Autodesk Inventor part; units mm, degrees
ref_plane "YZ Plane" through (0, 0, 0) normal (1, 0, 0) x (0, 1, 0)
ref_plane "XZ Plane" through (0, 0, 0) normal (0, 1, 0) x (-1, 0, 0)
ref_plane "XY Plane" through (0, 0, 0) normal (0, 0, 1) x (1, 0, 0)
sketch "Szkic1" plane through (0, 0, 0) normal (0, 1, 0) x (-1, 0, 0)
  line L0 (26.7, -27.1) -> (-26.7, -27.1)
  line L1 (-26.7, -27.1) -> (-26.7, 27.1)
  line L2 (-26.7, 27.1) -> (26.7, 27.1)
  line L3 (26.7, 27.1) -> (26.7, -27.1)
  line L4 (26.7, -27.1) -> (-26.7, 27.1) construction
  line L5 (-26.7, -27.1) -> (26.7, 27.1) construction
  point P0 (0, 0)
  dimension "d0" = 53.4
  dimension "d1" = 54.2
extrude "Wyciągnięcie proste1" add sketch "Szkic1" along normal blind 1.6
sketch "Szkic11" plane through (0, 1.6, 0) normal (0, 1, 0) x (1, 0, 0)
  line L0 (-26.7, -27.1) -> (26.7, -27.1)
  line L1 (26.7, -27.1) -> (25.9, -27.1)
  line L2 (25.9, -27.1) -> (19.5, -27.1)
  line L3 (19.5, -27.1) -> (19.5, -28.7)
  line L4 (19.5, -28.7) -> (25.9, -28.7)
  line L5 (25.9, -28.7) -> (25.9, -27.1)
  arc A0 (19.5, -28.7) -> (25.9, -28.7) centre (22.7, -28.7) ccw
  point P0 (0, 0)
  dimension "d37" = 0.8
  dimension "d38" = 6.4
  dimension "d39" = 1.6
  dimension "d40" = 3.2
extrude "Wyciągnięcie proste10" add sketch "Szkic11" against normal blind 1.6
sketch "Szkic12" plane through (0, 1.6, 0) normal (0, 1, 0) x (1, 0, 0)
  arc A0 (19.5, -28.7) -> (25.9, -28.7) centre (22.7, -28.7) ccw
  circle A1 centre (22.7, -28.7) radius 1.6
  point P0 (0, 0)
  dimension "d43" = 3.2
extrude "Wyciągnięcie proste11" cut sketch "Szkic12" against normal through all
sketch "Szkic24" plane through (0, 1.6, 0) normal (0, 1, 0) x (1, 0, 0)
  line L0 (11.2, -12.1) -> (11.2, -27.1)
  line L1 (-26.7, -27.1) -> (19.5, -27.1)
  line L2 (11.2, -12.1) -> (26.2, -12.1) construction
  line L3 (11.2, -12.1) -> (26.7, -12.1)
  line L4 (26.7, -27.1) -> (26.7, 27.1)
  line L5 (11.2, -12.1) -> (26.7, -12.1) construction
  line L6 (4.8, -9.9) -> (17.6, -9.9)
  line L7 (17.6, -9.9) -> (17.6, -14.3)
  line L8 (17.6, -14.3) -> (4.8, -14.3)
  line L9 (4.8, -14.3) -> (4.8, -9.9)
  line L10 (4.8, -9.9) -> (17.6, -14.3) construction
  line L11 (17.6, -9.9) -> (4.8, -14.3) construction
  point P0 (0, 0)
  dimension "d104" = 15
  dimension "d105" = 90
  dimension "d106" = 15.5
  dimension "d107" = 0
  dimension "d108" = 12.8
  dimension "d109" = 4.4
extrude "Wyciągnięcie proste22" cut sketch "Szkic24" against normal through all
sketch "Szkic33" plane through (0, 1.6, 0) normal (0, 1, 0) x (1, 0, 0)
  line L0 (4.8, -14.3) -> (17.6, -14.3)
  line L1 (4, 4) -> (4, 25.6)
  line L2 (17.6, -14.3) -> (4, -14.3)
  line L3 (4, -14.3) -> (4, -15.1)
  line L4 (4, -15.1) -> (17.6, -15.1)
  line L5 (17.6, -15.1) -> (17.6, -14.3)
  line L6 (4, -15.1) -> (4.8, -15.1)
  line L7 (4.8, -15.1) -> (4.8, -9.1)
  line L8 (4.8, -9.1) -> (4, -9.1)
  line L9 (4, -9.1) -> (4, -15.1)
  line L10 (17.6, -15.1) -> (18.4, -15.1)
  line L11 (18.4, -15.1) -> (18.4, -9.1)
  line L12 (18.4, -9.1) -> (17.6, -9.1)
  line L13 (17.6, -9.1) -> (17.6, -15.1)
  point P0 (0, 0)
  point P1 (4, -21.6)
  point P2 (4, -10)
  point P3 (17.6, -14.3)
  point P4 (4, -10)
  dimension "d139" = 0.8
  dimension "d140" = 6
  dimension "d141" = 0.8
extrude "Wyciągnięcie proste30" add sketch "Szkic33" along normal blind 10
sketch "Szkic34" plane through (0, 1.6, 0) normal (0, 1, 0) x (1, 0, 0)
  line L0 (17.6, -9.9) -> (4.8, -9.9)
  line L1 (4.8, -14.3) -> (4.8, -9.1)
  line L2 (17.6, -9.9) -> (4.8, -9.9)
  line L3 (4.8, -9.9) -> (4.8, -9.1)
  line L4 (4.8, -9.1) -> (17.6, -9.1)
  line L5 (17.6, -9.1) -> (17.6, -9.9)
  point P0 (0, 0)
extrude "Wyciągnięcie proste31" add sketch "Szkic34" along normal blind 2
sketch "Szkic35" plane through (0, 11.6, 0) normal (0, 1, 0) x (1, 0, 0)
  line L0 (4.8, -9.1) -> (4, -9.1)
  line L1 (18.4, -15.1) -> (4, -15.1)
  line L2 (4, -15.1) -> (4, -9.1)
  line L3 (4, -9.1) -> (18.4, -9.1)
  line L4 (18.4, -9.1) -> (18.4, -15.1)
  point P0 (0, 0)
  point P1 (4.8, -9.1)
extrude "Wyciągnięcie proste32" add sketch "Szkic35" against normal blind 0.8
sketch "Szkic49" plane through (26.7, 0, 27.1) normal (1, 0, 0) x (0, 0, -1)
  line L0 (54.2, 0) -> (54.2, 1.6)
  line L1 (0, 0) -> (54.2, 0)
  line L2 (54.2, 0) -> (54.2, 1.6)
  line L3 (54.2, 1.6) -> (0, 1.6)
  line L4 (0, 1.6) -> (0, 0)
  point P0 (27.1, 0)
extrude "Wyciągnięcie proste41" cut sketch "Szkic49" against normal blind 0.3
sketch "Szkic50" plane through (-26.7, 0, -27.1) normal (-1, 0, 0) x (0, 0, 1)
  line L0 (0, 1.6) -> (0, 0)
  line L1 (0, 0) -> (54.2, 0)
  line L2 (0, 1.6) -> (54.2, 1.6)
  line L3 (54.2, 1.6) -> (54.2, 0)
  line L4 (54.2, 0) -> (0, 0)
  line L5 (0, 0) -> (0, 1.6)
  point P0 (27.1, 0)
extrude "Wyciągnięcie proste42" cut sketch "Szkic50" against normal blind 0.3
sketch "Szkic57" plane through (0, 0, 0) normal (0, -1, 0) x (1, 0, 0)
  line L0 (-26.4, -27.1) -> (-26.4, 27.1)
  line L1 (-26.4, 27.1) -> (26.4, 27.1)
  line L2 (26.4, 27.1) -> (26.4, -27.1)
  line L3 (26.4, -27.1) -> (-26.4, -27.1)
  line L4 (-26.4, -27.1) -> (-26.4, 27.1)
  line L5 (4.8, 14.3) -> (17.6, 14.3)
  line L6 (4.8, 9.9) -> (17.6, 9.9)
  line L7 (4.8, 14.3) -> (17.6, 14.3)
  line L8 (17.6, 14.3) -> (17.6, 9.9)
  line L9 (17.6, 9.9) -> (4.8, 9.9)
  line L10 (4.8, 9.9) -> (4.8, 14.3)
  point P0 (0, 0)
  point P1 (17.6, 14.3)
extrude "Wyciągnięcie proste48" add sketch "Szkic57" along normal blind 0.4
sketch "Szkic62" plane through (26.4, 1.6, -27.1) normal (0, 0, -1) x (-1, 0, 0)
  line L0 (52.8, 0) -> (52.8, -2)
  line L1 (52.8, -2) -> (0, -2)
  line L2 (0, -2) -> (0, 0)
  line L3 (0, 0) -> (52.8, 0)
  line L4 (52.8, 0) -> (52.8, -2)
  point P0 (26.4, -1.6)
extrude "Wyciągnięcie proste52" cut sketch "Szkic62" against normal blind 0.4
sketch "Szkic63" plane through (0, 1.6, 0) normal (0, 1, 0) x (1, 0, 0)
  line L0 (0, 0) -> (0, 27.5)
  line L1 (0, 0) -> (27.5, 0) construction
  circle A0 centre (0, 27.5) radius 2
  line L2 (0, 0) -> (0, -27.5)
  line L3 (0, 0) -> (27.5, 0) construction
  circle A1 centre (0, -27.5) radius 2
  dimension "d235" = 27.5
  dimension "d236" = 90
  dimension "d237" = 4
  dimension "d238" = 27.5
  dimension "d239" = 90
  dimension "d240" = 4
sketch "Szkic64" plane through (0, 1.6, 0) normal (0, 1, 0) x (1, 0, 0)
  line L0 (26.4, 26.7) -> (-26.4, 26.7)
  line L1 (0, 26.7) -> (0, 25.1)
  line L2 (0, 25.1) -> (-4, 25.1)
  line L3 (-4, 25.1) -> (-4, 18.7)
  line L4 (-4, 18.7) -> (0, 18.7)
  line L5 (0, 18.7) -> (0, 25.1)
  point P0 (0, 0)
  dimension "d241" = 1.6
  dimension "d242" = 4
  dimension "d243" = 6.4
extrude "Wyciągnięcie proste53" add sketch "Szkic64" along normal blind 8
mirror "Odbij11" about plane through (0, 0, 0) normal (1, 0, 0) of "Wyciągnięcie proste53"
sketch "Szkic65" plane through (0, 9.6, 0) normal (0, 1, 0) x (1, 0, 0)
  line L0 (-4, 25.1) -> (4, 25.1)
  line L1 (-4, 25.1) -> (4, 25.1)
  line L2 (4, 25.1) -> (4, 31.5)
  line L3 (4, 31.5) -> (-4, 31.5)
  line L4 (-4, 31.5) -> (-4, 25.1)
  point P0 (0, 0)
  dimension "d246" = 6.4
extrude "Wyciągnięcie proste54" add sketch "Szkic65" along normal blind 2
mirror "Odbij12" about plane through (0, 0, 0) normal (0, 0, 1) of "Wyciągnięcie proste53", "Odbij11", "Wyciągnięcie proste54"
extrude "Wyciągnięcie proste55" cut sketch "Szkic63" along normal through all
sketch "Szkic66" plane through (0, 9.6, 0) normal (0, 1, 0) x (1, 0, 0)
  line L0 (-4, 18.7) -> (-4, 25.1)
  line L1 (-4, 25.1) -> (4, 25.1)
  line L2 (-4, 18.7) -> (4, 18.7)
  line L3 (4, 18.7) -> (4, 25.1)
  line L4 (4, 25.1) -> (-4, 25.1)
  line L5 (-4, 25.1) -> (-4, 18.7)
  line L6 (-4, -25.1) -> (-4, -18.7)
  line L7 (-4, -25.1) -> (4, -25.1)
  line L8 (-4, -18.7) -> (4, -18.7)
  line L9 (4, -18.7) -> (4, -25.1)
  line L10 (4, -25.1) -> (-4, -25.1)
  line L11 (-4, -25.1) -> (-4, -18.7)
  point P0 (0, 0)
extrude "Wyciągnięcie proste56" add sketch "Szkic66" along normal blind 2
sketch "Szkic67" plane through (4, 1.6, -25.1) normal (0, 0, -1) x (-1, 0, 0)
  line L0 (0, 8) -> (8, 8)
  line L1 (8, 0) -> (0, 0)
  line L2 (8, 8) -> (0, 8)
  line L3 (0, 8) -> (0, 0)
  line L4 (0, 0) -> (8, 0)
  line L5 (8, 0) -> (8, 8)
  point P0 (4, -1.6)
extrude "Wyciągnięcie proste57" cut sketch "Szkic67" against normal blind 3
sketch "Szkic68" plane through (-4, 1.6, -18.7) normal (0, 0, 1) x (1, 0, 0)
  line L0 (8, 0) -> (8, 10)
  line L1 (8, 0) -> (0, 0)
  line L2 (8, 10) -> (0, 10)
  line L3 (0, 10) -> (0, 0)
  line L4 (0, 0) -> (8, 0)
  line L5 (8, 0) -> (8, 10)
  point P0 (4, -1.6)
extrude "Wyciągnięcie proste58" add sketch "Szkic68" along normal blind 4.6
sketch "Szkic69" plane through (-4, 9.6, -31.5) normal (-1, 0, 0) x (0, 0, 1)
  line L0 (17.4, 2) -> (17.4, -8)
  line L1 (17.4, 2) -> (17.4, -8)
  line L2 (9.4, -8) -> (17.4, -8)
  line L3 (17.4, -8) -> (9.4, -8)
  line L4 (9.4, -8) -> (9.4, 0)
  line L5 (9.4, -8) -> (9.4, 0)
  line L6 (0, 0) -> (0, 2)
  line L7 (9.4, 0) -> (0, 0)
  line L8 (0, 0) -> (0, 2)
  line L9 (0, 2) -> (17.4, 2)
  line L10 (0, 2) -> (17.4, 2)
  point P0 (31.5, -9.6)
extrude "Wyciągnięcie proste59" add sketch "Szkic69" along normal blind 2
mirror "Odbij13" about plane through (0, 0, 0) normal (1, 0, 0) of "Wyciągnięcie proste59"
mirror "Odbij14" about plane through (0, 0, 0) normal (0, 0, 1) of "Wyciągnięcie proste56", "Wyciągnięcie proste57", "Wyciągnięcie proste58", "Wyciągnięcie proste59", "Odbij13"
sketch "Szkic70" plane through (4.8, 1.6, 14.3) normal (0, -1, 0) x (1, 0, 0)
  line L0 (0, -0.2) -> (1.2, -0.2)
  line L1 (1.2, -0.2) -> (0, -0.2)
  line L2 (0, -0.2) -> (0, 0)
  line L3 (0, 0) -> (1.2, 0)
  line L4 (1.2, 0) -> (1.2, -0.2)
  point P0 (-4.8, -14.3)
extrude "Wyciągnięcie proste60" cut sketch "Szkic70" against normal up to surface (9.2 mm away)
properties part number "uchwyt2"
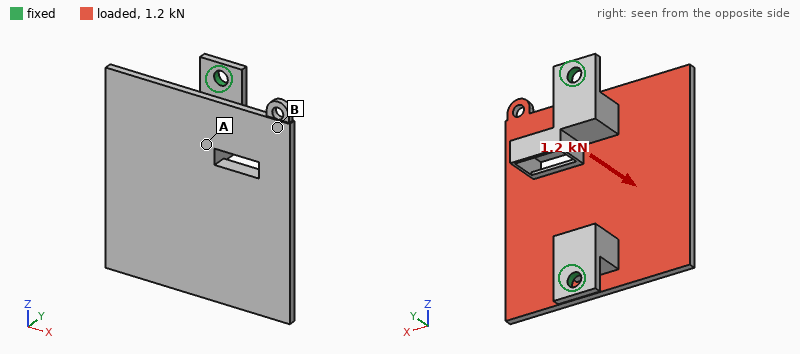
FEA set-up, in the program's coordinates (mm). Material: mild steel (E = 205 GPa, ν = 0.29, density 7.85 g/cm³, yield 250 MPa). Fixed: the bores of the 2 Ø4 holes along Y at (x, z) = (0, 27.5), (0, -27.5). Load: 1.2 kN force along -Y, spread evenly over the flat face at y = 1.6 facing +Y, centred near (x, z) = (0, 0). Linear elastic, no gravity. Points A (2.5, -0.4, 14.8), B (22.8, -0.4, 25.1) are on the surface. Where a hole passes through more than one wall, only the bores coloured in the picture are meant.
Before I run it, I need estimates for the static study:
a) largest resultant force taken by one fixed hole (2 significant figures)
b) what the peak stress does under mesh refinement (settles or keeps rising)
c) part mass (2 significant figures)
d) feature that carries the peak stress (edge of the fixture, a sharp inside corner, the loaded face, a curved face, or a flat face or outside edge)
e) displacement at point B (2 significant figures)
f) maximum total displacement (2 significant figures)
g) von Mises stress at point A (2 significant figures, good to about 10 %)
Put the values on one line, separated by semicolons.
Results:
820 N; keeps rising; 64 g; edge of the fixture; 0.034 mm; 0.14 mm; 32 MPa
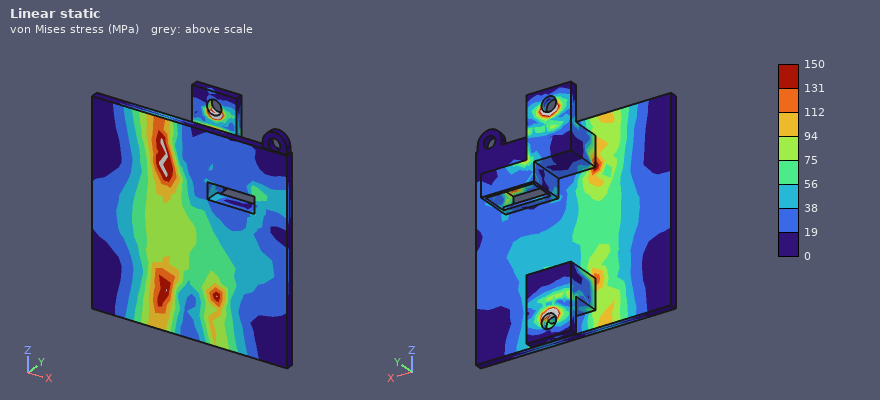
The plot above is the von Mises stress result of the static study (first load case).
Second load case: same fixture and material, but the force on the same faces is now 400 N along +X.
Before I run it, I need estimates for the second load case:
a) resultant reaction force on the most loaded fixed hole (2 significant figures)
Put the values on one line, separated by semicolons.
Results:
200 N
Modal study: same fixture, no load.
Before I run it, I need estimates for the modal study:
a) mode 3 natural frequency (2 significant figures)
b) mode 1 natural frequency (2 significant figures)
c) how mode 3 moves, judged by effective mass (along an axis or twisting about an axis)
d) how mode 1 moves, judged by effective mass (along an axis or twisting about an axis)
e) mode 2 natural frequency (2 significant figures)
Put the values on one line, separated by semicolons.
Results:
3400 Hz; 1500 Hz; along Y; along X; 3000 Hz
